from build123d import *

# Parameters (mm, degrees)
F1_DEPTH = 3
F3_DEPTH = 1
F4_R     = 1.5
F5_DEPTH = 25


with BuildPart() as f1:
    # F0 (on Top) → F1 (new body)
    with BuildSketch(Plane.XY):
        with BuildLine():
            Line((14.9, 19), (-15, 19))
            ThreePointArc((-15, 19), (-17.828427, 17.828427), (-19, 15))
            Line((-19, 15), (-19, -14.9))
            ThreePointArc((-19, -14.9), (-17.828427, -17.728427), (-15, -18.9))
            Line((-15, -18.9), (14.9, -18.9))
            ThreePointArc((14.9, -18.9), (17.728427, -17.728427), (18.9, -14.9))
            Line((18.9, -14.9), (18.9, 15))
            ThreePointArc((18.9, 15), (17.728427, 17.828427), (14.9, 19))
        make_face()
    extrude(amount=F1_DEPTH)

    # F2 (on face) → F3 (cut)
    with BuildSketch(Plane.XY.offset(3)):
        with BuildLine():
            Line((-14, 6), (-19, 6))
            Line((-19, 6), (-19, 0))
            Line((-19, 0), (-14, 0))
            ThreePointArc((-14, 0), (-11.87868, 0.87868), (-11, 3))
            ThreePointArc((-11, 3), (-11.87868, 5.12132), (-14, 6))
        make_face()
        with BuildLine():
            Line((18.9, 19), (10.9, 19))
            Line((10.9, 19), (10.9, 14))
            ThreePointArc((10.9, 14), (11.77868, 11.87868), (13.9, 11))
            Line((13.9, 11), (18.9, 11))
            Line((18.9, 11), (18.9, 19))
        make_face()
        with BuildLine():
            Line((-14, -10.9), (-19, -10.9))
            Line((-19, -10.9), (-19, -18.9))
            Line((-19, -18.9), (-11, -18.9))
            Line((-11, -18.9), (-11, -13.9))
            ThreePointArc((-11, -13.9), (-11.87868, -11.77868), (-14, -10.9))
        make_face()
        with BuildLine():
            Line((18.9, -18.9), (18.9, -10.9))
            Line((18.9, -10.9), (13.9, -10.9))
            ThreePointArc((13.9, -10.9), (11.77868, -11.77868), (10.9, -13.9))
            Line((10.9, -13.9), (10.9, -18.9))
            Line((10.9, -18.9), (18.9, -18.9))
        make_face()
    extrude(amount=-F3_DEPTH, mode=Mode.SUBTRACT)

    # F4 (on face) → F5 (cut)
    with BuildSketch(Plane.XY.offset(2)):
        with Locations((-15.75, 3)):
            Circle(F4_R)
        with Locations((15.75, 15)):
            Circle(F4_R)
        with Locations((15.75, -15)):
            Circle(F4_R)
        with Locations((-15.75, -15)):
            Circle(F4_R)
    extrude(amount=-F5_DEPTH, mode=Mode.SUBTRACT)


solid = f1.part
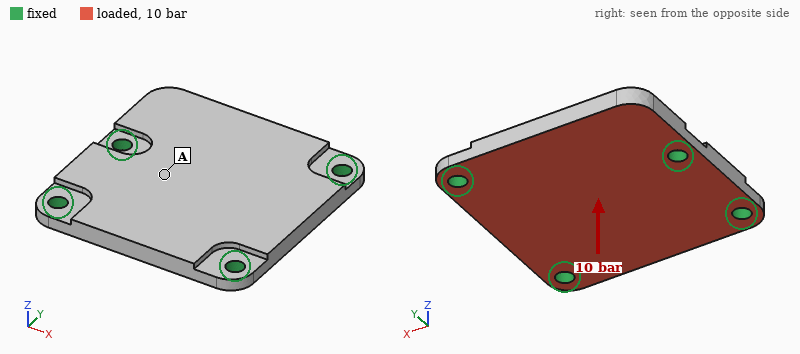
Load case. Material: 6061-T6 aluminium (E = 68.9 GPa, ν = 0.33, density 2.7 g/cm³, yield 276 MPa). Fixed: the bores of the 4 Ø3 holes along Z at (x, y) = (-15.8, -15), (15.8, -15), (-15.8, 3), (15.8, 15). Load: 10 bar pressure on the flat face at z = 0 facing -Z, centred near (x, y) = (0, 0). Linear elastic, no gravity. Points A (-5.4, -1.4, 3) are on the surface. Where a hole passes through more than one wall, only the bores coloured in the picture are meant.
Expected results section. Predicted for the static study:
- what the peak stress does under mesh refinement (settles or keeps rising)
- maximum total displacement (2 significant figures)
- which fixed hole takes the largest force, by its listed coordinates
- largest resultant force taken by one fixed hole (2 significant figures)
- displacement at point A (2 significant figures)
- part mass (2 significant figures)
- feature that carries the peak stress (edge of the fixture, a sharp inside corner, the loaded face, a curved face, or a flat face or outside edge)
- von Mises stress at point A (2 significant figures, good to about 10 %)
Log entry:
keeps rising
75 µm
(-15.8, 3)
570 N
30 µm
11 g
edge of the fixture
30 MPa
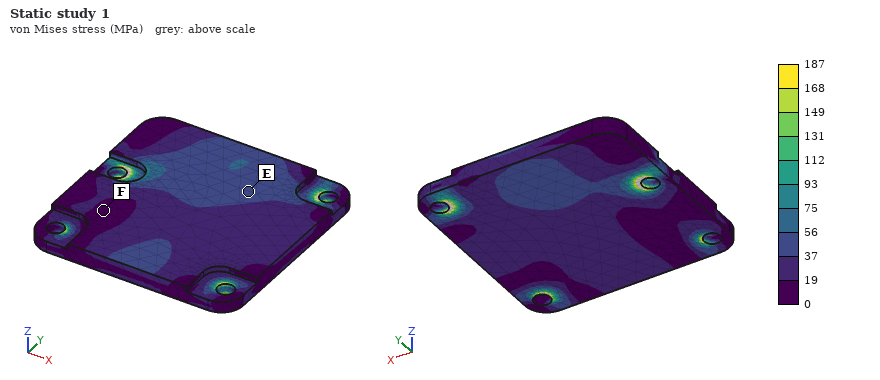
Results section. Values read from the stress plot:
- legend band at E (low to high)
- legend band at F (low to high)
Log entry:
37 to 56 MPa
0 to 19 MPa
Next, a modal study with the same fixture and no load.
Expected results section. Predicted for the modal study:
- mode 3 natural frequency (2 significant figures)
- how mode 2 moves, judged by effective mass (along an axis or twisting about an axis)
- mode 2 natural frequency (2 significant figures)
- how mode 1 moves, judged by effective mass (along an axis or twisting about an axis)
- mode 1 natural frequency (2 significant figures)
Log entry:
15 kHz
along Z
11 kHz
along Z
8200 Hz
